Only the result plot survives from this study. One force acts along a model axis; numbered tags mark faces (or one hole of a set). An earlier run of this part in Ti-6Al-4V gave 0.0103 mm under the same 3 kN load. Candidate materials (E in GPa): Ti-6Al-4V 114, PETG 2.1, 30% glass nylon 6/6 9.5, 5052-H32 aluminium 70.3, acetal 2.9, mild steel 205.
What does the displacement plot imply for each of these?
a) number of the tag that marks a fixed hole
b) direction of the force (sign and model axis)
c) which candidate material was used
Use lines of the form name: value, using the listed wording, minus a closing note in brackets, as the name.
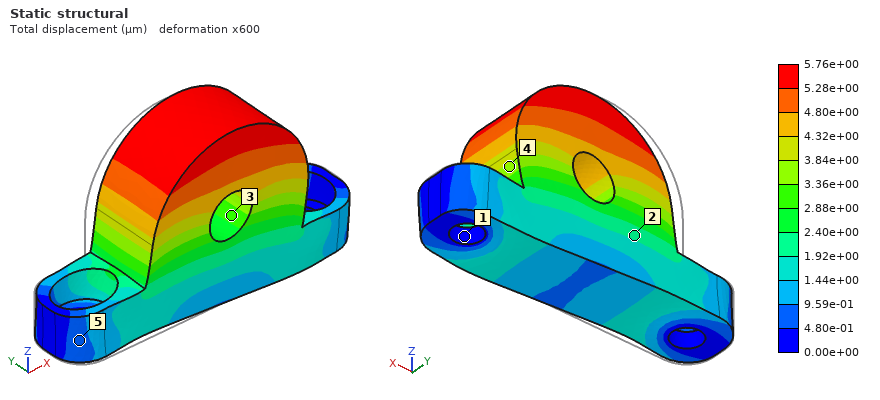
number of the tag that marks a fixed hole: 1
direction of the force: +X
which candidate material was used: mild steel
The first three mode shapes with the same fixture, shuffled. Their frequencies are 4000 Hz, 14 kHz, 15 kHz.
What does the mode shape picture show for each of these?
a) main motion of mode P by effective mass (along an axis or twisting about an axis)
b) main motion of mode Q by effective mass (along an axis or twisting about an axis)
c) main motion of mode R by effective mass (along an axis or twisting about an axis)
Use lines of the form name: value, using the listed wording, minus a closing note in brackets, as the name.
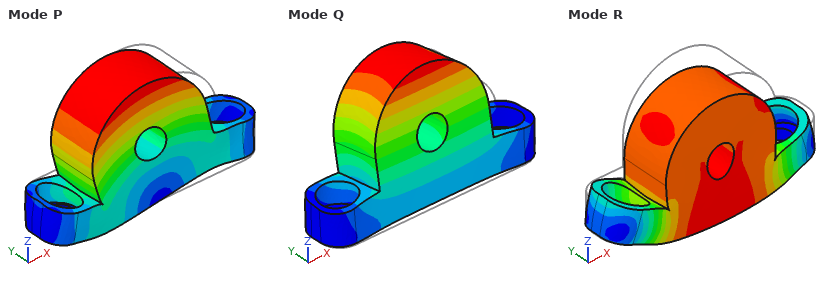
main motion of mode P by effective mass: along X
main motion of mode Q by effective mass: along Y
main motion of mode R by effective mass: along Z
